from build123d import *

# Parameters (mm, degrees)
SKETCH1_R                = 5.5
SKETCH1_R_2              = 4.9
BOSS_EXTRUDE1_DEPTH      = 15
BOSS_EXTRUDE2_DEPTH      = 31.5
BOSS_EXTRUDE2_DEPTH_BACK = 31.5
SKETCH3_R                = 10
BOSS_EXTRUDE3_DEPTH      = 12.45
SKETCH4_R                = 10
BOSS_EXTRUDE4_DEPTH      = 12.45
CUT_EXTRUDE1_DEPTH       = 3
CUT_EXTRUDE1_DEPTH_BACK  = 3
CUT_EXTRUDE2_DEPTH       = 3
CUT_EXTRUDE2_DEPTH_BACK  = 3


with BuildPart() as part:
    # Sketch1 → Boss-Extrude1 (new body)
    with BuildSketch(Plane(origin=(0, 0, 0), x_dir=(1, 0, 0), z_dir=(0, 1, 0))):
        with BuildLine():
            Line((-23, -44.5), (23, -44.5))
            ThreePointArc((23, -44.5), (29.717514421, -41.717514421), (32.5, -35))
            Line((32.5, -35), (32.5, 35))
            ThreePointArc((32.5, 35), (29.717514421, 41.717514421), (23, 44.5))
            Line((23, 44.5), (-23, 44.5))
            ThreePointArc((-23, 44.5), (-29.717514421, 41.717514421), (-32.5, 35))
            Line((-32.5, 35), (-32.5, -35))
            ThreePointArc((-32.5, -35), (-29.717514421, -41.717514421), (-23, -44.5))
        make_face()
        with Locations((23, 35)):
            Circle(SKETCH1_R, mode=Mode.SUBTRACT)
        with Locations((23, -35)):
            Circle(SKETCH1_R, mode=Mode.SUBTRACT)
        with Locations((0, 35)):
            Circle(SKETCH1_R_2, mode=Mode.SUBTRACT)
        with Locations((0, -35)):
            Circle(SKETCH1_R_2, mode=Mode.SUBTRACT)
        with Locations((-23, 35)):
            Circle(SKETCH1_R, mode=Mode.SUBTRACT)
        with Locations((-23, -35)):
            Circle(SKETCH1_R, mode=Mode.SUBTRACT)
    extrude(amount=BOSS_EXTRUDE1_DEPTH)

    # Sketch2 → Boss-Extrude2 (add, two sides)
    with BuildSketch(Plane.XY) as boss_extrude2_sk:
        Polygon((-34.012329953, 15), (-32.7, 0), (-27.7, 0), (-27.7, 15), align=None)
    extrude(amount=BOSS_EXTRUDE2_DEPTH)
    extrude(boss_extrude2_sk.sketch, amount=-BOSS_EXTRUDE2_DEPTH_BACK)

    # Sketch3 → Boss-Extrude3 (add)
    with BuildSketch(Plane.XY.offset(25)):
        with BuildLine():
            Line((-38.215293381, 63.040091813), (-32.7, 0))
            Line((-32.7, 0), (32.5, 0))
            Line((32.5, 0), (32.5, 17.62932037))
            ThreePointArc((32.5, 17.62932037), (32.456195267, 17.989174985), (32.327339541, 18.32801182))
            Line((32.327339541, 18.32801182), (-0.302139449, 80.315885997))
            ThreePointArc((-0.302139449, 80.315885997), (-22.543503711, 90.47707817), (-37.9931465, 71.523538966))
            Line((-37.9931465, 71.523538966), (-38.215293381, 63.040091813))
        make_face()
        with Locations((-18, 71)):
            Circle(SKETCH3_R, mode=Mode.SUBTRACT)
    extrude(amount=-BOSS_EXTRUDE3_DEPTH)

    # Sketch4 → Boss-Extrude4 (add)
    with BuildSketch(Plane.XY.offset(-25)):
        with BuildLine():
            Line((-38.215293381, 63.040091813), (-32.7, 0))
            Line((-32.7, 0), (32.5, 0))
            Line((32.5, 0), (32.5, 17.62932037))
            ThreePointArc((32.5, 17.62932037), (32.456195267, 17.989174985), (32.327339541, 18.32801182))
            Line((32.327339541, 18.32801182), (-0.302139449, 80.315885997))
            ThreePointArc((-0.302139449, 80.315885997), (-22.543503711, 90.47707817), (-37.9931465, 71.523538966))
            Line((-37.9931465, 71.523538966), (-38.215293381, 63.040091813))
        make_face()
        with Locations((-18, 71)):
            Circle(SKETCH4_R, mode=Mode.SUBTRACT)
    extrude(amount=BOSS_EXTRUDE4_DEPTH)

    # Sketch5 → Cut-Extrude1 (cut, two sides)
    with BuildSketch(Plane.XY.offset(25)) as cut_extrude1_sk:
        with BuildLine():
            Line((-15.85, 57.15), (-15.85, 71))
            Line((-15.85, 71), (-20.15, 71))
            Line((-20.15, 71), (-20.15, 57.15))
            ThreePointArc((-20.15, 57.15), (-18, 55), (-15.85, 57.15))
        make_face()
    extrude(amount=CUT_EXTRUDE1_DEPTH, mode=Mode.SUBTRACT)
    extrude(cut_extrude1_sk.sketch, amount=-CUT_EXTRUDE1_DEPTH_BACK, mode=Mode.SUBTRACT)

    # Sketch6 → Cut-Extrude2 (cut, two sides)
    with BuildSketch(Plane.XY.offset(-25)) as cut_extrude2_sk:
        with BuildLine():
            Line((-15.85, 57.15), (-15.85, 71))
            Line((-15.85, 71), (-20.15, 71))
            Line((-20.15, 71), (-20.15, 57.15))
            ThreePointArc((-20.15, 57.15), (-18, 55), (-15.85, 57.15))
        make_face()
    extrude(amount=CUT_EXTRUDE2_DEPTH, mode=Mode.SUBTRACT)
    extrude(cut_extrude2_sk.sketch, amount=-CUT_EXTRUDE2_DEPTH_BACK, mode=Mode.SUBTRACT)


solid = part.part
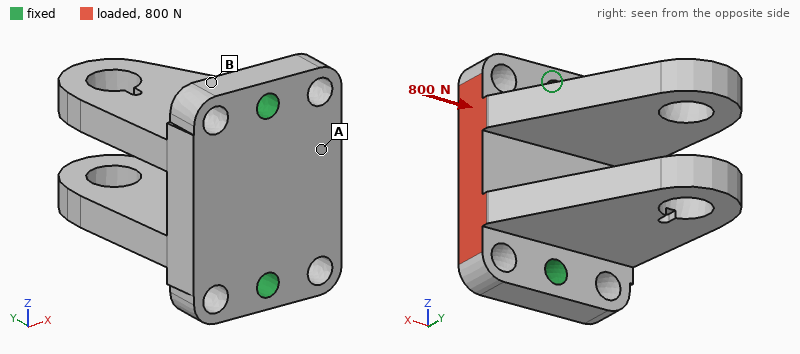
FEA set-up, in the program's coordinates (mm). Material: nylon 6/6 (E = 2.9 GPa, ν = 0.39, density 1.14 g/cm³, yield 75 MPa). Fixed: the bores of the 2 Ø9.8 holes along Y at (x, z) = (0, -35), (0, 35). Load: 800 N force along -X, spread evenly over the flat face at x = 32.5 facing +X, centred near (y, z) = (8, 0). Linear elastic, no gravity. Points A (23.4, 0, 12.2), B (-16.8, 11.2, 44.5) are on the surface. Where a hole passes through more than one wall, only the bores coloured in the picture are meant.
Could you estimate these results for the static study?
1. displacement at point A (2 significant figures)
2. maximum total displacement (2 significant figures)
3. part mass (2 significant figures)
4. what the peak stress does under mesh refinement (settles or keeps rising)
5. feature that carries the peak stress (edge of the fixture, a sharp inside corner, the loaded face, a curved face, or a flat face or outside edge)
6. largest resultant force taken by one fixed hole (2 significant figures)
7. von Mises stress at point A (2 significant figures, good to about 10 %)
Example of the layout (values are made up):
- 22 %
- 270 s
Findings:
- 13 µm
- 16 µm
- 190 g
- keeps rising
- edge of the fixture
- 410 N
- 0.66 MPa
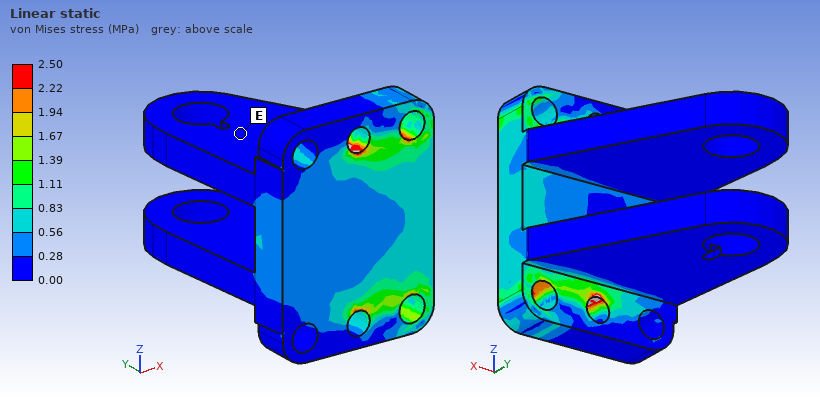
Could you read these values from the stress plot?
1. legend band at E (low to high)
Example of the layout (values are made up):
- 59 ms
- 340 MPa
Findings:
- 0.00 to 0.28 MPa
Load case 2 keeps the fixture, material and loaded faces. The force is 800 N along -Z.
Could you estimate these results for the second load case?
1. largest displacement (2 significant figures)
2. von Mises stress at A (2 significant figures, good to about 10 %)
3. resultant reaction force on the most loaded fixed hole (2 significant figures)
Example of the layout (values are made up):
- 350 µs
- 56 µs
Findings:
- 31 µm
- 1.6 MPa
- 530 N
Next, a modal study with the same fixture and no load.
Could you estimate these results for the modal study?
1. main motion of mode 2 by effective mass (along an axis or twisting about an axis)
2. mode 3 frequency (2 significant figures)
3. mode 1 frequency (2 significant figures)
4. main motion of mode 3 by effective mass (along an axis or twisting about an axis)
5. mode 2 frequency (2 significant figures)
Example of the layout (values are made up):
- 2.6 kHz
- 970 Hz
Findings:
- along Z
- 790 Hz
- 620 Hz
- along X
- 690 Hz
